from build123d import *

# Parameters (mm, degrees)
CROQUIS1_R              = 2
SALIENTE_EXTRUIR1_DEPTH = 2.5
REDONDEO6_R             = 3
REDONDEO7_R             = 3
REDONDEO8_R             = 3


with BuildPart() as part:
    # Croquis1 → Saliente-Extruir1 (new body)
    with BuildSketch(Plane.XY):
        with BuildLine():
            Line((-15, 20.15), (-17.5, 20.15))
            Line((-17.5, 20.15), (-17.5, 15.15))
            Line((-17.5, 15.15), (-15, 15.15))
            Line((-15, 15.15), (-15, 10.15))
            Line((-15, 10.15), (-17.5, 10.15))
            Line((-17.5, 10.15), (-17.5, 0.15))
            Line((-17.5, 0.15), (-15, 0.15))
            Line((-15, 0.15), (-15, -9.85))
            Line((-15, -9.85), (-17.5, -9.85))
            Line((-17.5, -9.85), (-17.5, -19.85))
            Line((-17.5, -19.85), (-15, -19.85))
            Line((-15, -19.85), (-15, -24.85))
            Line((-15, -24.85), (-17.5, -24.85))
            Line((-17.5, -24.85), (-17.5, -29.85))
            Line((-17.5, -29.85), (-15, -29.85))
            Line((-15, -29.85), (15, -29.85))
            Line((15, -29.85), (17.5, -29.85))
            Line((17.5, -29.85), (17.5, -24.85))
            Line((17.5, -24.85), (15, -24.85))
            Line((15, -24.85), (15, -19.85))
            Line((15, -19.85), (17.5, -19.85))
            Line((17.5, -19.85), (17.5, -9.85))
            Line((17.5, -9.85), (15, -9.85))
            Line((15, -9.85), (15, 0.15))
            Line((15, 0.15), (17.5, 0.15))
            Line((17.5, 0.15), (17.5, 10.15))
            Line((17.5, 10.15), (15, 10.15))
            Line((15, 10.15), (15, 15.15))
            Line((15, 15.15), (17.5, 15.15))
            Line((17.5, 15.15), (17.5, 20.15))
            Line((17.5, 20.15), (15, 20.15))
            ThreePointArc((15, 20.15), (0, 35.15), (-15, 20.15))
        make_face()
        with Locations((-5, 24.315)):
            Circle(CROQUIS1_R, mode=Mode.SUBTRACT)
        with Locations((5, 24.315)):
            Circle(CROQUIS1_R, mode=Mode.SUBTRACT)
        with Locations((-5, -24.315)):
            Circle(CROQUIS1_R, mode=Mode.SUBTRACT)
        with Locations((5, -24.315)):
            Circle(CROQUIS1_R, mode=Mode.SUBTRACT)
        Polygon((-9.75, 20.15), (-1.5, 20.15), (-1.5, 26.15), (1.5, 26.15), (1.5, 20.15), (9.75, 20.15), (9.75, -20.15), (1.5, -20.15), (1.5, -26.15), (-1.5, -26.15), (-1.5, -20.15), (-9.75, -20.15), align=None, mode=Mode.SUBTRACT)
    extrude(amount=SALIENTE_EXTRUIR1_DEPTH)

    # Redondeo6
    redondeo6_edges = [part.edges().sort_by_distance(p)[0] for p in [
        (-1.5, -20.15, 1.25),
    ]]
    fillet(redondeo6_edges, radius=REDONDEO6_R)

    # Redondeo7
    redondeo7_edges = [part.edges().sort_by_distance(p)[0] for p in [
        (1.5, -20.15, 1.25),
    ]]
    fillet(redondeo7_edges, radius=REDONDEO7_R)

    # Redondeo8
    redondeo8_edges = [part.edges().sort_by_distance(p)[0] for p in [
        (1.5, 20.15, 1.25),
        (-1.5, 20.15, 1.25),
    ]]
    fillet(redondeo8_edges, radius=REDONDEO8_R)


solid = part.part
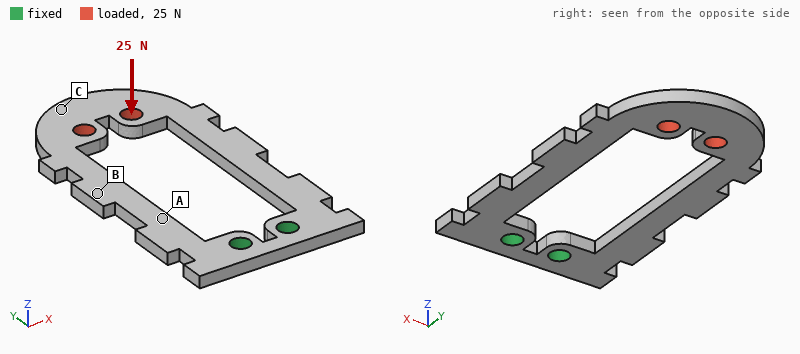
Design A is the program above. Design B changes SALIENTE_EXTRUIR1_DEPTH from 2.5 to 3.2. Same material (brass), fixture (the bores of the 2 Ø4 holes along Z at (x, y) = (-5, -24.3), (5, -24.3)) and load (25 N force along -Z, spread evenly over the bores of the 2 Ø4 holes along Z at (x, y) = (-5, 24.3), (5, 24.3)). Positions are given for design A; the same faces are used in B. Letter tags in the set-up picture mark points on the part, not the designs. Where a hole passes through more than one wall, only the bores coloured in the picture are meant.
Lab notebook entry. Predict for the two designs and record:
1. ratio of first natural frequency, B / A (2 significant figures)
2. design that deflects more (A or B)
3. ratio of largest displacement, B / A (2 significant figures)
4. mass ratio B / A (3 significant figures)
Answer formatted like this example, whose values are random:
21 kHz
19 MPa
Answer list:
1.3
A
0.49
1.28
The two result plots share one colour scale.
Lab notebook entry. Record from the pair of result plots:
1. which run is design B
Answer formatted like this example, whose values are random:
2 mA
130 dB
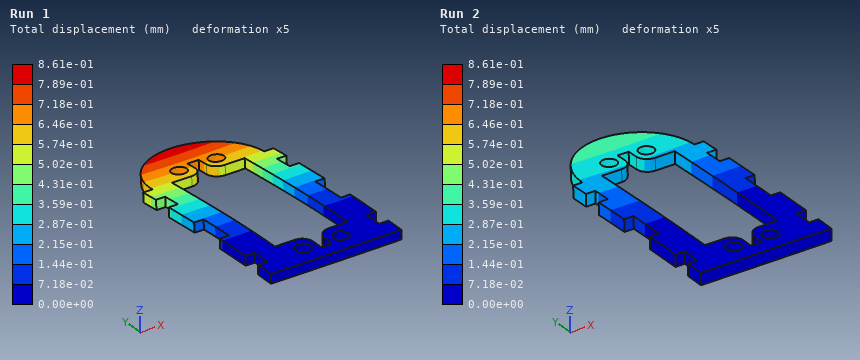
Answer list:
Run 2
